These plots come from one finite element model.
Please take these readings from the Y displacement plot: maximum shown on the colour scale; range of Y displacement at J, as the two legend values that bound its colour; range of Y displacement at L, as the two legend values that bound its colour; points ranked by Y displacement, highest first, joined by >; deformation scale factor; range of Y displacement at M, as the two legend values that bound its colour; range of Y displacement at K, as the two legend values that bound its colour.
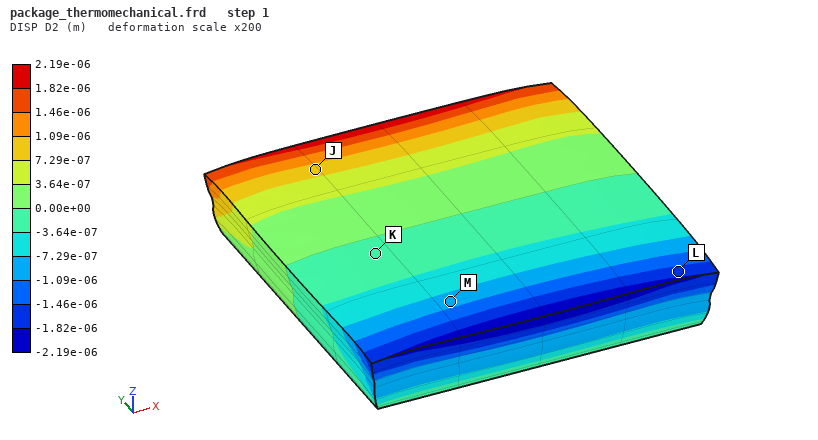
2.19e-06 m
7.29e-07 to 1.09e-06 m
-1.82e-06 to -1.46e-06 m
J > K > M > L
200
-1.09e-06 to -7.29e-07 m
-3.64e-07 to 0.00e+00 m
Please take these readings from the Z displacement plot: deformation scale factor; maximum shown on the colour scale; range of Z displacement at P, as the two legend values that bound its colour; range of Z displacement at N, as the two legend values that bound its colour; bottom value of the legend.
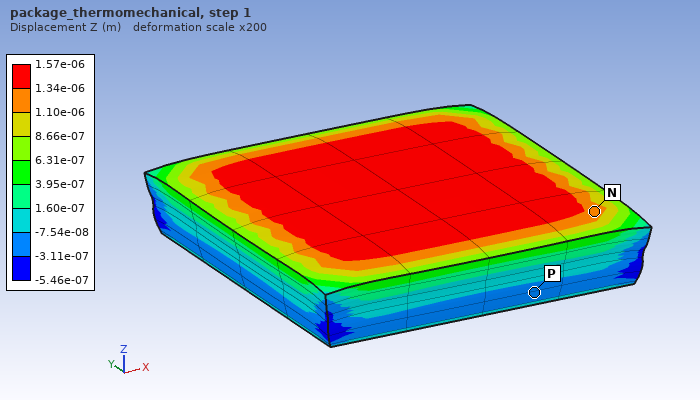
200
1.57e-06 m
-3.11e-07 to -7.54e-08 m
1.10e-06 to 1.34e-06 m
-5.46e-07 m
